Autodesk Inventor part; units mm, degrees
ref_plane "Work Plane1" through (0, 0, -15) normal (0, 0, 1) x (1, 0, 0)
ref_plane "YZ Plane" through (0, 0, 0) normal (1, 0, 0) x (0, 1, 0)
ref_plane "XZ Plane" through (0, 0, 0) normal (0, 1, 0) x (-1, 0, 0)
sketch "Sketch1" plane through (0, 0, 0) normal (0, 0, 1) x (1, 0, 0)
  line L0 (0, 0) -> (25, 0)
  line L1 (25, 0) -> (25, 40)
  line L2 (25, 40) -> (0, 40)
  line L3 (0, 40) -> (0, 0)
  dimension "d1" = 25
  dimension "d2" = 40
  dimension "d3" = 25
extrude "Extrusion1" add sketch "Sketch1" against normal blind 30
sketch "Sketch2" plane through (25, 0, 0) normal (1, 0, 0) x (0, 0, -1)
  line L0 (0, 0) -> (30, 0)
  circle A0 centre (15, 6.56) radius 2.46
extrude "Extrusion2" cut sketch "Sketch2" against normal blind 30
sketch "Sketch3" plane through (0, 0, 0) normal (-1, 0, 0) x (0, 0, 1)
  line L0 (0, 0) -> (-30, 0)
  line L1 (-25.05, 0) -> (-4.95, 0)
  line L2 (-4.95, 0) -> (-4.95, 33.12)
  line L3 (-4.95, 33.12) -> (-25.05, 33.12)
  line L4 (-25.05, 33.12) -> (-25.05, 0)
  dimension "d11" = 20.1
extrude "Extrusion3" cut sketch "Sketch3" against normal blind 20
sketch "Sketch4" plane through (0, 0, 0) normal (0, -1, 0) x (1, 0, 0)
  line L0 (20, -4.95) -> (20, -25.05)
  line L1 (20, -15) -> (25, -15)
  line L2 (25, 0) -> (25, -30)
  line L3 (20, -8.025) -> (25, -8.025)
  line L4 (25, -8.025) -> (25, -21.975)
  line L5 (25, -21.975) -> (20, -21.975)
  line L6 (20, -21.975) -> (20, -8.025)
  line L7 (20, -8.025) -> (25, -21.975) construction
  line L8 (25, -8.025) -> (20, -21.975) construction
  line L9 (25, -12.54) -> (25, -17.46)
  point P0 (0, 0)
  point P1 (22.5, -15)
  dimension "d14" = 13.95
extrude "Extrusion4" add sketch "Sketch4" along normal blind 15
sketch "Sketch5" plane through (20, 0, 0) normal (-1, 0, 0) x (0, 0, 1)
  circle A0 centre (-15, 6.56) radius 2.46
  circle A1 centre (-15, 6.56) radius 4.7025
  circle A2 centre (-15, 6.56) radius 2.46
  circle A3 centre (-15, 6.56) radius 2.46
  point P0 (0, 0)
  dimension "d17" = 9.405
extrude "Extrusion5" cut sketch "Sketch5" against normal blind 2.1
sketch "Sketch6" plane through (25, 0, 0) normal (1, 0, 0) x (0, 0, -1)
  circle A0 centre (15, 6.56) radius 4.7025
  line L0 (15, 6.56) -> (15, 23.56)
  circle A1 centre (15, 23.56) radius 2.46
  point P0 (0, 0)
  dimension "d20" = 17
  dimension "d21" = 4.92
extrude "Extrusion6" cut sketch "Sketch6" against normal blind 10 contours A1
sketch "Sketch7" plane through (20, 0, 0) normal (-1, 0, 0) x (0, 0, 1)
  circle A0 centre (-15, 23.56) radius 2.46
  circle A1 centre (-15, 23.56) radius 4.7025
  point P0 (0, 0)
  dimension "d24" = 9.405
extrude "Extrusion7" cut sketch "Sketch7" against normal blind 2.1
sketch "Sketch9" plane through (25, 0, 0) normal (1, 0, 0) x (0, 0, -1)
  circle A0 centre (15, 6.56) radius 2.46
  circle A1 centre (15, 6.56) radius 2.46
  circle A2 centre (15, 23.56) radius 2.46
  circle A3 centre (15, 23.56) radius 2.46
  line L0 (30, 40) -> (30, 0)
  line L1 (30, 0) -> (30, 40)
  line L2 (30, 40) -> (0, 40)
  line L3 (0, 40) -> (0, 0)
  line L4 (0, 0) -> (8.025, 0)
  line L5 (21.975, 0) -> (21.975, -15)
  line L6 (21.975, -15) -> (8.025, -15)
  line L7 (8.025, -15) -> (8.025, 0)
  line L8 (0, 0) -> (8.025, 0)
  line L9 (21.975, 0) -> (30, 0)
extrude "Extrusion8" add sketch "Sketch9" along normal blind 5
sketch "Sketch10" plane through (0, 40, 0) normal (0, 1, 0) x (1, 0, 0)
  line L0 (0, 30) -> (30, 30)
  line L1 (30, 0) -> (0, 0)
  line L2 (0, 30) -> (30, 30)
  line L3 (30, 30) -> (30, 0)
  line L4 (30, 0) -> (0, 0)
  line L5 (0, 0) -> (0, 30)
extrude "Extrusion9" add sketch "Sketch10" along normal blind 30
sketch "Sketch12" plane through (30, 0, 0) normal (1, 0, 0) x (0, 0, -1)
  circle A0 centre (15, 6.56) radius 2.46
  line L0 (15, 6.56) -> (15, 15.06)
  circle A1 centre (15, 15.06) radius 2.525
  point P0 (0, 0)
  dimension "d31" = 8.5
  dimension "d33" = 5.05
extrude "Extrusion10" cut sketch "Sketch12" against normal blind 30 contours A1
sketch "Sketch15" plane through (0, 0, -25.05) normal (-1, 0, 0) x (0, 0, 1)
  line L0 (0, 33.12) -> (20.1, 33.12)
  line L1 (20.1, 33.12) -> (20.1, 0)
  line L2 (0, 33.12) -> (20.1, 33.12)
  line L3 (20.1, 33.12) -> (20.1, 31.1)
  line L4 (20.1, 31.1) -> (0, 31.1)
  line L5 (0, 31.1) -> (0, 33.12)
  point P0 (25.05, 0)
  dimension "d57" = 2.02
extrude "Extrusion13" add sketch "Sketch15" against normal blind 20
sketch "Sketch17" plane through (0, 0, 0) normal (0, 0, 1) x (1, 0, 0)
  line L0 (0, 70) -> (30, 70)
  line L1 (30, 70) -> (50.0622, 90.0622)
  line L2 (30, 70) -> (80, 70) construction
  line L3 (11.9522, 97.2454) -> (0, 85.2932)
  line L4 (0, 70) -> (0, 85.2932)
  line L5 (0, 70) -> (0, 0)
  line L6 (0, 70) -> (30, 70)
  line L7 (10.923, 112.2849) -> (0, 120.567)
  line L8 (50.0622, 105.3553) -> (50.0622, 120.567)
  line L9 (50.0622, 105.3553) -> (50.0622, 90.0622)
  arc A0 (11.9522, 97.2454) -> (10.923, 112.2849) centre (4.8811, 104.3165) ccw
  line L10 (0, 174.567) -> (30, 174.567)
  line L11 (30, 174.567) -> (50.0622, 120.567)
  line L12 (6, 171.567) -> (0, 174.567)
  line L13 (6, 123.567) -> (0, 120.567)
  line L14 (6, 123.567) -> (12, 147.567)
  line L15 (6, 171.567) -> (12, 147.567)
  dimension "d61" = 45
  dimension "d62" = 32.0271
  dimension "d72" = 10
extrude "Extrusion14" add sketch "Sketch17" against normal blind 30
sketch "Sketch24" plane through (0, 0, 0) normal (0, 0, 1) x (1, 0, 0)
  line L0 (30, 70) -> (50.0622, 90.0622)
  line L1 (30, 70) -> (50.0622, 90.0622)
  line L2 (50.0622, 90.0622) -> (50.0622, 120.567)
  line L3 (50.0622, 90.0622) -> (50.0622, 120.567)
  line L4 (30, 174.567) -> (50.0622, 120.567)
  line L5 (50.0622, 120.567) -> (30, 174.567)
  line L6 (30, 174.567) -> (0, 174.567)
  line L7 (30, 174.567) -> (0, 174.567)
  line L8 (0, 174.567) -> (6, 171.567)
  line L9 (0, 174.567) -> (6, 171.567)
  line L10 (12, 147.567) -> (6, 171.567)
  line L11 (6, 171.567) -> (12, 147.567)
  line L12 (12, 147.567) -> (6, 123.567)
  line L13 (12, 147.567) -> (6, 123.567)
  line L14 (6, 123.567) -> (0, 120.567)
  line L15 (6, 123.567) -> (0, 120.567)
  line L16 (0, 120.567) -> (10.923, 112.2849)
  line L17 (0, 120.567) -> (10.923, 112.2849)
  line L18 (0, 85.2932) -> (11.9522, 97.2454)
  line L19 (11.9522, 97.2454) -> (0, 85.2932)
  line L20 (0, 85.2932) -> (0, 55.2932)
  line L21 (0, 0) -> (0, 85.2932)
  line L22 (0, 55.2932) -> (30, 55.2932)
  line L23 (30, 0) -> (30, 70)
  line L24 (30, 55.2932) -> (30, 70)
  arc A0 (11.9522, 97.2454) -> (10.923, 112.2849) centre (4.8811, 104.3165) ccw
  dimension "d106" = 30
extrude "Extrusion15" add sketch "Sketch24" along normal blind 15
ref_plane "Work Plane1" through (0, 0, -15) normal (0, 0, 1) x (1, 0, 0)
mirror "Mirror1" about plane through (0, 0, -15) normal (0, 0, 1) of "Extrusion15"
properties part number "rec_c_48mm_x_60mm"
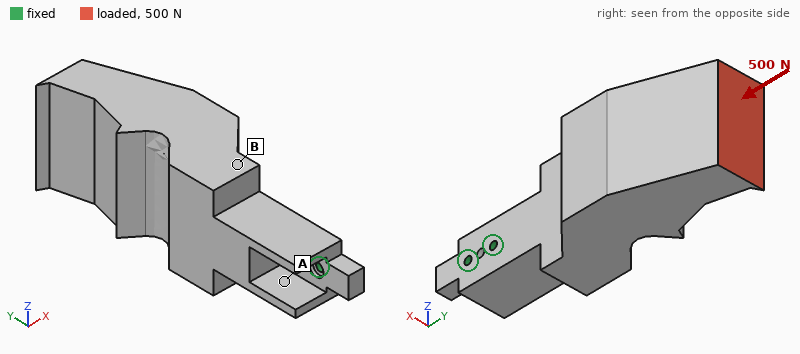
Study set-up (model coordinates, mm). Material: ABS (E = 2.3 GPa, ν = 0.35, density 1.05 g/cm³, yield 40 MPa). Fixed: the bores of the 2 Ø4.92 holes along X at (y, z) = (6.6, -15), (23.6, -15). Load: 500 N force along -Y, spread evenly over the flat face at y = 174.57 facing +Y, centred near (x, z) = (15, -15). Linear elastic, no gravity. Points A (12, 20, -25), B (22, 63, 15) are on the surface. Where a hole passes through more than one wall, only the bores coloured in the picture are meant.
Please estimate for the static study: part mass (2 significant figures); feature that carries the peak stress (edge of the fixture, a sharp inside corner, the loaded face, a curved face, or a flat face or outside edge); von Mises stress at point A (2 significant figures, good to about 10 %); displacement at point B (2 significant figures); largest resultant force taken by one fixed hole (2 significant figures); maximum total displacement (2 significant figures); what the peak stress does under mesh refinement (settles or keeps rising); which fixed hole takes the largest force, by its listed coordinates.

300 g
edge of the fixture
1.8 MPa
0.14 mm
380 N
0.62 mm
keeps rising
(23.6, -15)
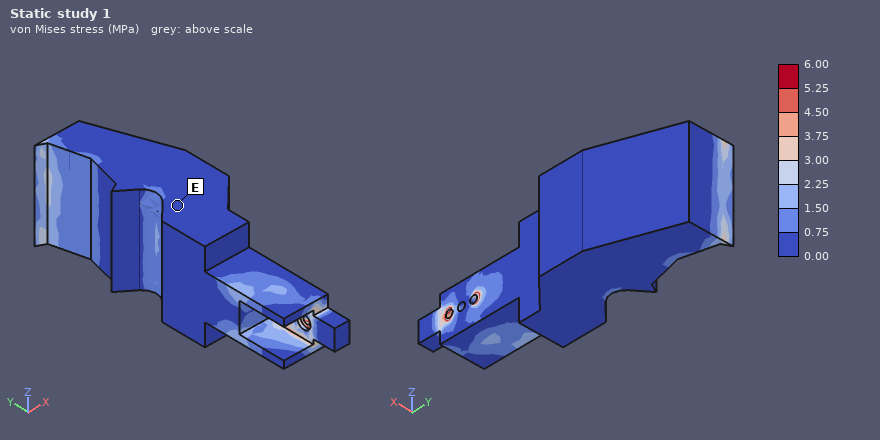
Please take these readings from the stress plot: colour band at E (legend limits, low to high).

0.00 to 0.75 MPa
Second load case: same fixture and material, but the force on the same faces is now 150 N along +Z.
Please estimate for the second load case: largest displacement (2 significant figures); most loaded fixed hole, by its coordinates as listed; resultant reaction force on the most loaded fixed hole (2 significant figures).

2.2 mm
(23.6, -15)
1.1 kN
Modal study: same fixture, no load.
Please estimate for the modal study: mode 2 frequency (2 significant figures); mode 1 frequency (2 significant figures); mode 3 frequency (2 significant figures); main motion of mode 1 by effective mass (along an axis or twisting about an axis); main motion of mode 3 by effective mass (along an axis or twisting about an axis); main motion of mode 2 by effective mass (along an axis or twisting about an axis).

130 Hz
110 Hz
350 Hz
along X
twisting about Y
along Z
